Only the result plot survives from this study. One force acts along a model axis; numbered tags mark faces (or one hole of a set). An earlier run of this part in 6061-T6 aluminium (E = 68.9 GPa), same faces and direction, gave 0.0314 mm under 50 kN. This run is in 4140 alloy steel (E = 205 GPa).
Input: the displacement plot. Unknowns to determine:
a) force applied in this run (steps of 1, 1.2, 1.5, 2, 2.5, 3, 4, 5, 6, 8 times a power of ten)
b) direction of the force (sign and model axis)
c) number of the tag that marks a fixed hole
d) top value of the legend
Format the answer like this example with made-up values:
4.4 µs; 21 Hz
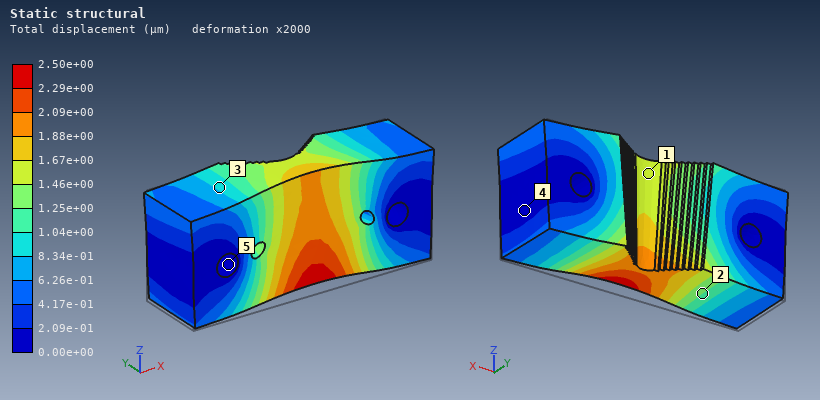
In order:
12 kN; +Z; 5; 2.50e+00 µm
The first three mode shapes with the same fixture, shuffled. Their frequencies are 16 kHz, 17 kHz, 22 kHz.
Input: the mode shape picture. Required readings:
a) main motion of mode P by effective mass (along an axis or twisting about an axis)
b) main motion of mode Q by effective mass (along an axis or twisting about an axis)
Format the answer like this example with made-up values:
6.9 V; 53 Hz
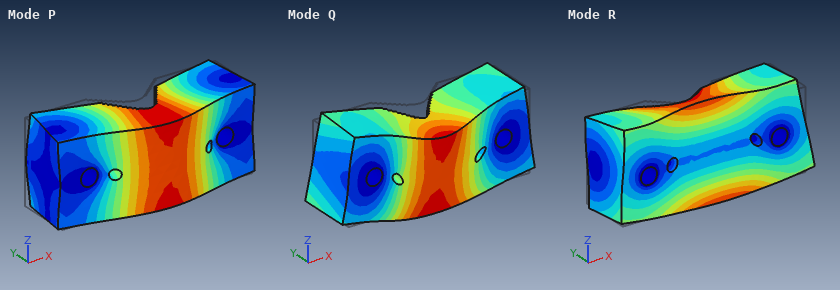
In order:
along Y; along Z
